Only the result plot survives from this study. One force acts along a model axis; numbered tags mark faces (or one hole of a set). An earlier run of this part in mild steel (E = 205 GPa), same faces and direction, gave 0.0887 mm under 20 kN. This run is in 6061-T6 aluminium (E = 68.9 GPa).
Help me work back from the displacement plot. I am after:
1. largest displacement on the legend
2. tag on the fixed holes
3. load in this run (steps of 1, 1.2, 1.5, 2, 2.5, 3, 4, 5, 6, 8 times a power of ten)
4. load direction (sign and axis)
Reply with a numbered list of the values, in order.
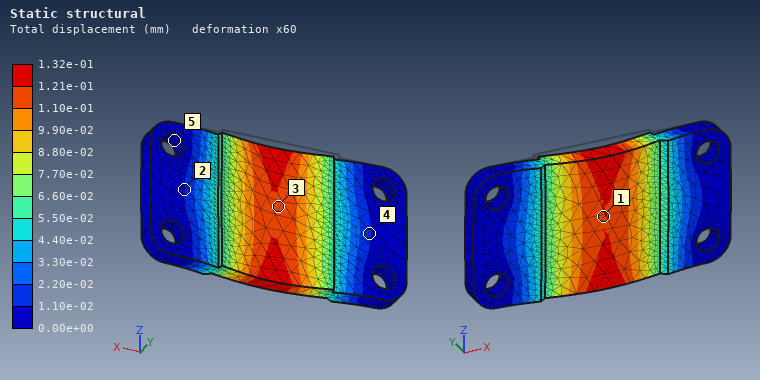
1. 1.32e-01 mm
2. 5
3. 10 kN
4. -Y
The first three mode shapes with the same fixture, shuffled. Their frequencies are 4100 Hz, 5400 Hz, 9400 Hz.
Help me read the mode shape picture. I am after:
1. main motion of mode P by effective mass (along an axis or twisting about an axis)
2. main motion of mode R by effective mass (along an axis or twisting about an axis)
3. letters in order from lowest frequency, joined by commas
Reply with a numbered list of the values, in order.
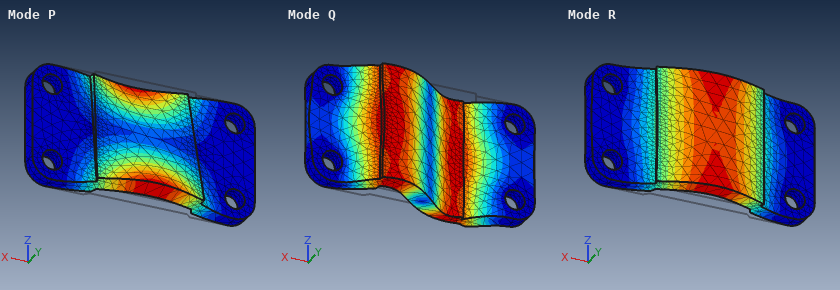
1. twisting about X
2. along Y
3. R, P, Q
